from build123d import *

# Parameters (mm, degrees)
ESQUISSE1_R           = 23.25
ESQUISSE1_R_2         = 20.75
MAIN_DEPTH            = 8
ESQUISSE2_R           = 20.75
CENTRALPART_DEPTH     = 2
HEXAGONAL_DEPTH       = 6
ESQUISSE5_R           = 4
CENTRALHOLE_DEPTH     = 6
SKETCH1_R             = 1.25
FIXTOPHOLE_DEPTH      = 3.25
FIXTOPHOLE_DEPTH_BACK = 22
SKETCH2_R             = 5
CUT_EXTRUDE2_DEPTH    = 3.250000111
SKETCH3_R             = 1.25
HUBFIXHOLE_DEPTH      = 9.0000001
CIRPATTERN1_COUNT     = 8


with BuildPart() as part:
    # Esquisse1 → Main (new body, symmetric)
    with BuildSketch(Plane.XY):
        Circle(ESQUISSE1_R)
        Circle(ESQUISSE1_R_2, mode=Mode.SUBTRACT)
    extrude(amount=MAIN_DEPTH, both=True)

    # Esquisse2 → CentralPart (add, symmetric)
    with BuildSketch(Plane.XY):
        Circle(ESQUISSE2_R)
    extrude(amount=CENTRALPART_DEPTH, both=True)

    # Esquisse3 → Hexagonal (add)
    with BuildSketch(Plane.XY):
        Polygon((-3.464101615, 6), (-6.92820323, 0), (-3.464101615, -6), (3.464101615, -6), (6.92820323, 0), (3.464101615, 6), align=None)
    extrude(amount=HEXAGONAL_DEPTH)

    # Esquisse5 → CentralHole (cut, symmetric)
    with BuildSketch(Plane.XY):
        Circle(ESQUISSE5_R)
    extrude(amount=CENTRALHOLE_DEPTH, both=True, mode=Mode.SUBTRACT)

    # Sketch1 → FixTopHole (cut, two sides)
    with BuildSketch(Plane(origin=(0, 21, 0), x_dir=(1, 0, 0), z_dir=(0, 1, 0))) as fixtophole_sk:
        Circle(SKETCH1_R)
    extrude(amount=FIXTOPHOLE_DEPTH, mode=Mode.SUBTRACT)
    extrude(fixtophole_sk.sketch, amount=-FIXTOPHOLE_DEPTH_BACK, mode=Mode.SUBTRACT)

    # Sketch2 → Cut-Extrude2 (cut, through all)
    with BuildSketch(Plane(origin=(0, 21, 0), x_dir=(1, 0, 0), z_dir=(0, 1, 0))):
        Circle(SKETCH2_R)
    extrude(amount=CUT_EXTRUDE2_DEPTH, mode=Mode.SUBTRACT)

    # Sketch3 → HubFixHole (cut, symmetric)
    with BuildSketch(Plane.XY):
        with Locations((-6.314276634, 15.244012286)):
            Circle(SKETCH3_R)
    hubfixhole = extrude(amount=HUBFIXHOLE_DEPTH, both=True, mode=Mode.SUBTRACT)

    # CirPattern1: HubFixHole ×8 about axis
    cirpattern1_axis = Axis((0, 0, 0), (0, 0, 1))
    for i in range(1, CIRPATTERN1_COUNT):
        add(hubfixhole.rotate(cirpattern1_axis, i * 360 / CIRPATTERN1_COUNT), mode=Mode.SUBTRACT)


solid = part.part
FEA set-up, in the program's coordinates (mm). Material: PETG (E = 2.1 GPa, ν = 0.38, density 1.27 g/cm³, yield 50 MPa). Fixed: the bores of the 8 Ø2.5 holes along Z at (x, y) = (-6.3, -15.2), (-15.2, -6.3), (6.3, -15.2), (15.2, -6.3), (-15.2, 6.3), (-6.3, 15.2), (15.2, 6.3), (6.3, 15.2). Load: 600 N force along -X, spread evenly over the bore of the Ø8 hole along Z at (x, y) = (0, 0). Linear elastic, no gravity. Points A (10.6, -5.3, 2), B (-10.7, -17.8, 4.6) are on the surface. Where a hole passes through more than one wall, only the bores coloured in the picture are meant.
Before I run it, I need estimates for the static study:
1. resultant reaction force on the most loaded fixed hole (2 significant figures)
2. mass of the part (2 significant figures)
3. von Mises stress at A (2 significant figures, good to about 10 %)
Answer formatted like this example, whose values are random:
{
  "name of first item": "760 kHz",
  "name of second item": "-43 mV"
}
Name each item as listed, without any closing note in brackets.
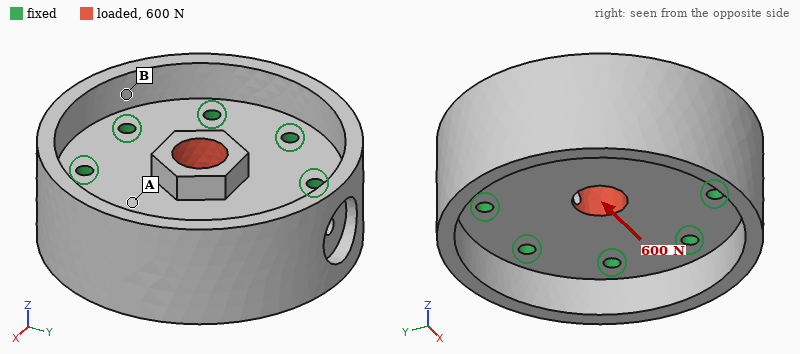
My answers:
{
  "resultant reaction force on the most loaded fixed hole": "120 N",
  "mass of the part": "13 g",
  "von Mises stress at A": "4.3 MPa"
}
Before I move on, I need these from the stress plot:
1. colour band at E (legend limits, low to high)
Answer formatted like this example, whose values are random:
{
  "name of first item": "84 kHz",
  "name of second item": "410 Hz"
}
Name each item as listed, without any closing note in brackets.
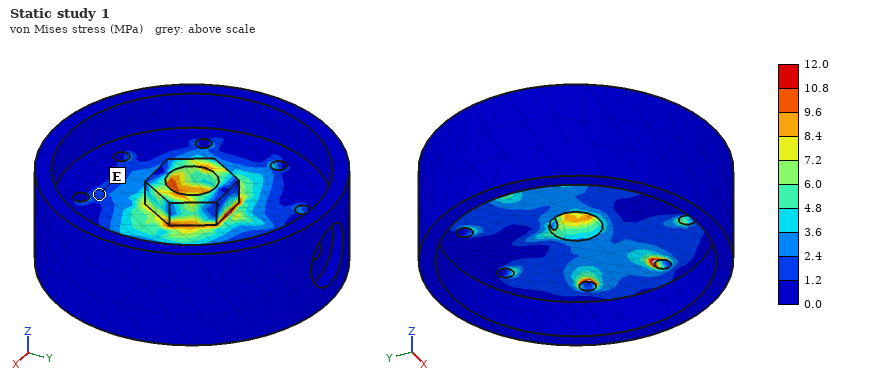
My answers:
{
  "colour band at E": "1.2 to 2.4 MPa"
}
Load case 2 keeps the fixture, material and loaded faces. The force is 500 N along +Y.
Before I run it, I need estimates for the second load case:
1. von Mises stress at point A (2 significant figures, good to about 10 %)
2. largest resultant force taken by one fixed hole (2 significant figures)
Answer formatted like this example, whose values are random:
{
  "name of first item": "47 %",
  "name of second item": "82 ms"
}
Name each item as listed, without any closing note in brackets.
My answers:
{
  "von Mises stress at point A": "1.9 MPa",
  "largest resultant force taken by one fixed hole": "100 N"
}
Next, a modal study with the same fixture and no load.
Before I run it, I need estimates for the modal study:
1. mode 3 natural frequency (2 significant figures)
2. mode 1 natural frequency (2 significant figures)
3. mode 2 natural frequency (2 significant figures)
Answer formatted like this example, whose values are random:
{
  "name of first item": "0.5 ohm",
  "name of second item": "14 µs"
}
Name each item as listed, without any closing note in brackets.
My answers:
{
  "mode 3 natural frequency": "6500 Hz",
  "mode 1 natural frequency": "5500 Hz",
  "mode 2 natural frequency": "5600 Hz"
}
